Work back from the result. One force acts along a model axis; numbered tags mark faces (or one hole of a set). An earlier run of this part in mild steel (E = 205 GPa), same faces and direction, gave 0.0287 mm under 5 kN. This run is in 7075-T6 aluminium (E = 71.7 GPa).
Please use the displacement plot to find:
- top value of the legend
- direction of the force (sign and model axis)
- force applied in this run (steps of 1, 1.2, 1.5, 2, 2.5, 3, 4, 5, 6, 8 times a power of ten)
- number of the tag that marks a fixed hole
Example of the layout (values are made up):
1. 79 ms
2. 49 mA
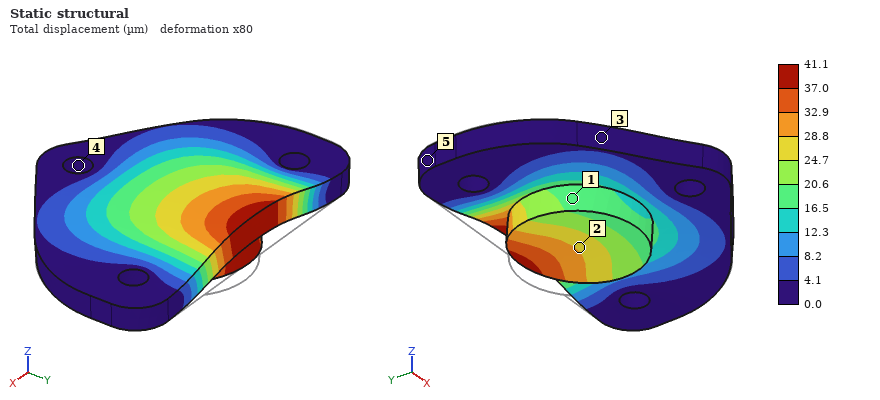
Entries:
1. 41.1 µm
2. +Z
3. 2.5 kN
4. 4
